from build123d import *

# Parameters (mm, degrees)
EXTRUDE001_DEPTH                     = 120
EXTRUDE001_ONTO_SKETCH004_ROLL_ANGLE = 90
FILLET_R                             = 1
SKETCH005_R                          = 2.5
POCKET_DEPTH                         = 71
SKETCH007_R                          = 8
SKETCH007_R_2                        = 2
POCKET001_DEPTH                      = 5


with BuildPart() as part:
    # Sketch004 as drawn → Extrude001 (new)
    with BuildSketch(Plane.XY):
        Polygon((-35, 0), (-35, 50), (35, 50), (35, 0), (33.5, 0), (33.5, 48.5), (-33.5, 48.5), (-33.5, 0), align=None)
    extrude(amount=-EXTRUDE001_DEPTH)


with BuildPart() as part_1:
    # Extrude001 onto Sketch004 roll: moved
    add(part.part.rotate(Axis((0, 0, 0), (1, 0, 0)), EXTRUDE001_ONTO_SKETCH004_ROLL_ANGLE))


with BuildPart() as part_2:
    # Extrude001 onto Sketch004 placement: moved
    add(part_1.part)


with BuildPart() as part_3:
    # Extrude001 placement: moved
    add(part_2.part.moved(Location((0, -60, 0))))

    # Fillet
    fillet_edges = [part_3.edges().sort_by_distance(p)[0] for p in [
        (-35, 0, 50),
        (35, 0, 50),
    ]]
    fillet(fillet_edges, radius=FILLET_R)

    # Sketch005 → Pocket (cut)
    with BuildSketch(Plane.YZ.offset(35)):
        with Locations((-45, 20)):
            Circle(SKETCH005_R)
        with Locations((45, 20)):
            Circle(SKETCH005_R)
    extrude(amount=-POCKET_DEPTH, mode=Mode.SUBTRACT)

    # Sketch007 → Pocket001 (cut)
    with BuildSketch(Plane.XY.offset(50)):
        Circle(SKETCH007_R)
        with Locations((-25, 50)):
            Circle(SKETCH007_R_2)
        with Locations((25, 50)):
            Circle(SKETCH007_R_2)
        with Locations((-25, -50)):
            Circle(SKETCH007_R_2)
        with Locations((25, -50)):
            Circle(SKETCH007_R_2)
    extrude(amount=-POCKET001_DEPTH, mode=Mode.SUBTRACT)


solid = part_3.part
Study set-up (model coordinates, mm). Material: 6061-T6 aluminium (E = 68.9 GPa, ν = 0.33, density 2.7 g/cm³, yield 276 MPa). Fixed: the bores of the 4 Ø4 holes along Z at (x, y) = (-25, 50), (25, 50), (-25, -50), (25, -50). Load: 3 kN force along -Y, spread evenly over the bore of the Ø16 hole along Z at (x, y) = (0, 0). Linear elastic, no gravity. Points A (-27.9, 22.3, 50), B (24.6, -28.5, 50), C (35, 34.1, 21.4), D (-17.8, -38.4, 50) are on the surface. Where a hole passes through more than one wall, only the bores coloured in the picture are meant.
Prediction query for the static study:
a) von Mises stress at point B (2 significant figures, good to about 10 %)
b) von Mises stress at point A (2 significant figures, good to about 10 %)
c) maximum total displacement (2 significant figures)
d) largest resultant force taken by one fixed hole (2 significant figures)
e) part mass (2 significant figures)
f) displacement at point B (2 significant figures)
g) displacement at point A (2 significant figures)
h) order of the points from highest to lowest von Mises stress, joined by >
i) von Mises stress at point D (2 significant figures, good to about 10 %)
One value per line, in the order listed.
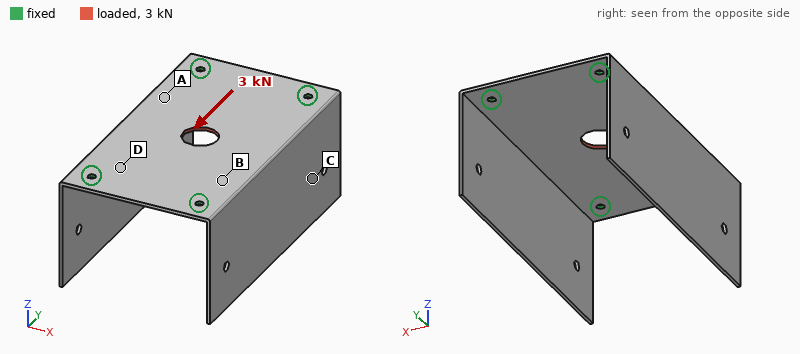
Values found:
16 MPa
10 MPa
20 µm
770 N
80 g
7.0 µm
7.4 µm
D > B > A > C
23 MPa
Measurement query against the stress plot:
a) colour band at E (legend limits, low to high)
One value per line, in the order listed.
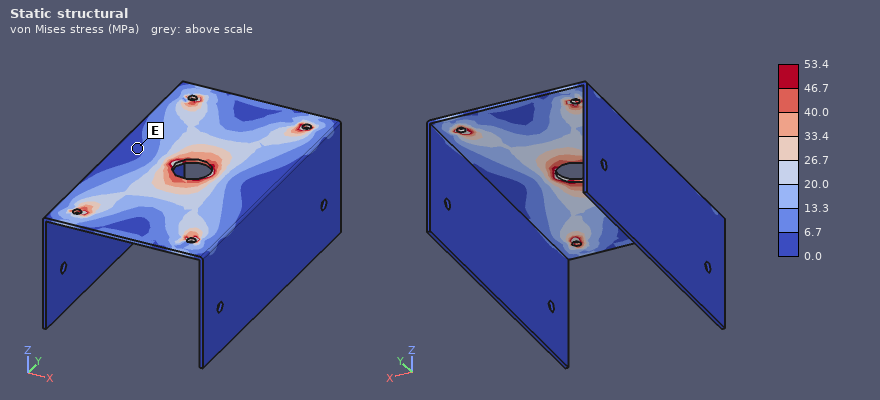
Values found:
0.0 to 6.7 MPa
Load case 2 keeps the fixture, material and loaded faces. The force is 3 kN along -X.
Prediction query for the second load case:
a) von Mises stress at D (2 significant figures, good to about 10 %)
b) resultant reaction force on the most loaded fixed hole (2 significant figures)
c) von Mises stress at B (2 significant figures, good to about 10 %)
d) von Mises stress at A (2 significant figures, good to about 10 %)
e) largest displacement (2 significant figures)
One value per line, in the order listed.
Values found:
31 MPa
900 N
22 MPa
19 MPa
39 µm
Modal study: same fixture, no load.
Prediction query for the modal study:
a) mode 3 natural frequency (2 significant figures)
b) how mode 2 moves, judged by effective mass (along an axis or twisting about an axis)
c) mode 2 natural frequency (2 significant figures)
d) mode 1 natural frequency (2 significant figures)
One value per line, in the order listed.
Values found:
600 Hz
along X
380 Hz
350 Hz
